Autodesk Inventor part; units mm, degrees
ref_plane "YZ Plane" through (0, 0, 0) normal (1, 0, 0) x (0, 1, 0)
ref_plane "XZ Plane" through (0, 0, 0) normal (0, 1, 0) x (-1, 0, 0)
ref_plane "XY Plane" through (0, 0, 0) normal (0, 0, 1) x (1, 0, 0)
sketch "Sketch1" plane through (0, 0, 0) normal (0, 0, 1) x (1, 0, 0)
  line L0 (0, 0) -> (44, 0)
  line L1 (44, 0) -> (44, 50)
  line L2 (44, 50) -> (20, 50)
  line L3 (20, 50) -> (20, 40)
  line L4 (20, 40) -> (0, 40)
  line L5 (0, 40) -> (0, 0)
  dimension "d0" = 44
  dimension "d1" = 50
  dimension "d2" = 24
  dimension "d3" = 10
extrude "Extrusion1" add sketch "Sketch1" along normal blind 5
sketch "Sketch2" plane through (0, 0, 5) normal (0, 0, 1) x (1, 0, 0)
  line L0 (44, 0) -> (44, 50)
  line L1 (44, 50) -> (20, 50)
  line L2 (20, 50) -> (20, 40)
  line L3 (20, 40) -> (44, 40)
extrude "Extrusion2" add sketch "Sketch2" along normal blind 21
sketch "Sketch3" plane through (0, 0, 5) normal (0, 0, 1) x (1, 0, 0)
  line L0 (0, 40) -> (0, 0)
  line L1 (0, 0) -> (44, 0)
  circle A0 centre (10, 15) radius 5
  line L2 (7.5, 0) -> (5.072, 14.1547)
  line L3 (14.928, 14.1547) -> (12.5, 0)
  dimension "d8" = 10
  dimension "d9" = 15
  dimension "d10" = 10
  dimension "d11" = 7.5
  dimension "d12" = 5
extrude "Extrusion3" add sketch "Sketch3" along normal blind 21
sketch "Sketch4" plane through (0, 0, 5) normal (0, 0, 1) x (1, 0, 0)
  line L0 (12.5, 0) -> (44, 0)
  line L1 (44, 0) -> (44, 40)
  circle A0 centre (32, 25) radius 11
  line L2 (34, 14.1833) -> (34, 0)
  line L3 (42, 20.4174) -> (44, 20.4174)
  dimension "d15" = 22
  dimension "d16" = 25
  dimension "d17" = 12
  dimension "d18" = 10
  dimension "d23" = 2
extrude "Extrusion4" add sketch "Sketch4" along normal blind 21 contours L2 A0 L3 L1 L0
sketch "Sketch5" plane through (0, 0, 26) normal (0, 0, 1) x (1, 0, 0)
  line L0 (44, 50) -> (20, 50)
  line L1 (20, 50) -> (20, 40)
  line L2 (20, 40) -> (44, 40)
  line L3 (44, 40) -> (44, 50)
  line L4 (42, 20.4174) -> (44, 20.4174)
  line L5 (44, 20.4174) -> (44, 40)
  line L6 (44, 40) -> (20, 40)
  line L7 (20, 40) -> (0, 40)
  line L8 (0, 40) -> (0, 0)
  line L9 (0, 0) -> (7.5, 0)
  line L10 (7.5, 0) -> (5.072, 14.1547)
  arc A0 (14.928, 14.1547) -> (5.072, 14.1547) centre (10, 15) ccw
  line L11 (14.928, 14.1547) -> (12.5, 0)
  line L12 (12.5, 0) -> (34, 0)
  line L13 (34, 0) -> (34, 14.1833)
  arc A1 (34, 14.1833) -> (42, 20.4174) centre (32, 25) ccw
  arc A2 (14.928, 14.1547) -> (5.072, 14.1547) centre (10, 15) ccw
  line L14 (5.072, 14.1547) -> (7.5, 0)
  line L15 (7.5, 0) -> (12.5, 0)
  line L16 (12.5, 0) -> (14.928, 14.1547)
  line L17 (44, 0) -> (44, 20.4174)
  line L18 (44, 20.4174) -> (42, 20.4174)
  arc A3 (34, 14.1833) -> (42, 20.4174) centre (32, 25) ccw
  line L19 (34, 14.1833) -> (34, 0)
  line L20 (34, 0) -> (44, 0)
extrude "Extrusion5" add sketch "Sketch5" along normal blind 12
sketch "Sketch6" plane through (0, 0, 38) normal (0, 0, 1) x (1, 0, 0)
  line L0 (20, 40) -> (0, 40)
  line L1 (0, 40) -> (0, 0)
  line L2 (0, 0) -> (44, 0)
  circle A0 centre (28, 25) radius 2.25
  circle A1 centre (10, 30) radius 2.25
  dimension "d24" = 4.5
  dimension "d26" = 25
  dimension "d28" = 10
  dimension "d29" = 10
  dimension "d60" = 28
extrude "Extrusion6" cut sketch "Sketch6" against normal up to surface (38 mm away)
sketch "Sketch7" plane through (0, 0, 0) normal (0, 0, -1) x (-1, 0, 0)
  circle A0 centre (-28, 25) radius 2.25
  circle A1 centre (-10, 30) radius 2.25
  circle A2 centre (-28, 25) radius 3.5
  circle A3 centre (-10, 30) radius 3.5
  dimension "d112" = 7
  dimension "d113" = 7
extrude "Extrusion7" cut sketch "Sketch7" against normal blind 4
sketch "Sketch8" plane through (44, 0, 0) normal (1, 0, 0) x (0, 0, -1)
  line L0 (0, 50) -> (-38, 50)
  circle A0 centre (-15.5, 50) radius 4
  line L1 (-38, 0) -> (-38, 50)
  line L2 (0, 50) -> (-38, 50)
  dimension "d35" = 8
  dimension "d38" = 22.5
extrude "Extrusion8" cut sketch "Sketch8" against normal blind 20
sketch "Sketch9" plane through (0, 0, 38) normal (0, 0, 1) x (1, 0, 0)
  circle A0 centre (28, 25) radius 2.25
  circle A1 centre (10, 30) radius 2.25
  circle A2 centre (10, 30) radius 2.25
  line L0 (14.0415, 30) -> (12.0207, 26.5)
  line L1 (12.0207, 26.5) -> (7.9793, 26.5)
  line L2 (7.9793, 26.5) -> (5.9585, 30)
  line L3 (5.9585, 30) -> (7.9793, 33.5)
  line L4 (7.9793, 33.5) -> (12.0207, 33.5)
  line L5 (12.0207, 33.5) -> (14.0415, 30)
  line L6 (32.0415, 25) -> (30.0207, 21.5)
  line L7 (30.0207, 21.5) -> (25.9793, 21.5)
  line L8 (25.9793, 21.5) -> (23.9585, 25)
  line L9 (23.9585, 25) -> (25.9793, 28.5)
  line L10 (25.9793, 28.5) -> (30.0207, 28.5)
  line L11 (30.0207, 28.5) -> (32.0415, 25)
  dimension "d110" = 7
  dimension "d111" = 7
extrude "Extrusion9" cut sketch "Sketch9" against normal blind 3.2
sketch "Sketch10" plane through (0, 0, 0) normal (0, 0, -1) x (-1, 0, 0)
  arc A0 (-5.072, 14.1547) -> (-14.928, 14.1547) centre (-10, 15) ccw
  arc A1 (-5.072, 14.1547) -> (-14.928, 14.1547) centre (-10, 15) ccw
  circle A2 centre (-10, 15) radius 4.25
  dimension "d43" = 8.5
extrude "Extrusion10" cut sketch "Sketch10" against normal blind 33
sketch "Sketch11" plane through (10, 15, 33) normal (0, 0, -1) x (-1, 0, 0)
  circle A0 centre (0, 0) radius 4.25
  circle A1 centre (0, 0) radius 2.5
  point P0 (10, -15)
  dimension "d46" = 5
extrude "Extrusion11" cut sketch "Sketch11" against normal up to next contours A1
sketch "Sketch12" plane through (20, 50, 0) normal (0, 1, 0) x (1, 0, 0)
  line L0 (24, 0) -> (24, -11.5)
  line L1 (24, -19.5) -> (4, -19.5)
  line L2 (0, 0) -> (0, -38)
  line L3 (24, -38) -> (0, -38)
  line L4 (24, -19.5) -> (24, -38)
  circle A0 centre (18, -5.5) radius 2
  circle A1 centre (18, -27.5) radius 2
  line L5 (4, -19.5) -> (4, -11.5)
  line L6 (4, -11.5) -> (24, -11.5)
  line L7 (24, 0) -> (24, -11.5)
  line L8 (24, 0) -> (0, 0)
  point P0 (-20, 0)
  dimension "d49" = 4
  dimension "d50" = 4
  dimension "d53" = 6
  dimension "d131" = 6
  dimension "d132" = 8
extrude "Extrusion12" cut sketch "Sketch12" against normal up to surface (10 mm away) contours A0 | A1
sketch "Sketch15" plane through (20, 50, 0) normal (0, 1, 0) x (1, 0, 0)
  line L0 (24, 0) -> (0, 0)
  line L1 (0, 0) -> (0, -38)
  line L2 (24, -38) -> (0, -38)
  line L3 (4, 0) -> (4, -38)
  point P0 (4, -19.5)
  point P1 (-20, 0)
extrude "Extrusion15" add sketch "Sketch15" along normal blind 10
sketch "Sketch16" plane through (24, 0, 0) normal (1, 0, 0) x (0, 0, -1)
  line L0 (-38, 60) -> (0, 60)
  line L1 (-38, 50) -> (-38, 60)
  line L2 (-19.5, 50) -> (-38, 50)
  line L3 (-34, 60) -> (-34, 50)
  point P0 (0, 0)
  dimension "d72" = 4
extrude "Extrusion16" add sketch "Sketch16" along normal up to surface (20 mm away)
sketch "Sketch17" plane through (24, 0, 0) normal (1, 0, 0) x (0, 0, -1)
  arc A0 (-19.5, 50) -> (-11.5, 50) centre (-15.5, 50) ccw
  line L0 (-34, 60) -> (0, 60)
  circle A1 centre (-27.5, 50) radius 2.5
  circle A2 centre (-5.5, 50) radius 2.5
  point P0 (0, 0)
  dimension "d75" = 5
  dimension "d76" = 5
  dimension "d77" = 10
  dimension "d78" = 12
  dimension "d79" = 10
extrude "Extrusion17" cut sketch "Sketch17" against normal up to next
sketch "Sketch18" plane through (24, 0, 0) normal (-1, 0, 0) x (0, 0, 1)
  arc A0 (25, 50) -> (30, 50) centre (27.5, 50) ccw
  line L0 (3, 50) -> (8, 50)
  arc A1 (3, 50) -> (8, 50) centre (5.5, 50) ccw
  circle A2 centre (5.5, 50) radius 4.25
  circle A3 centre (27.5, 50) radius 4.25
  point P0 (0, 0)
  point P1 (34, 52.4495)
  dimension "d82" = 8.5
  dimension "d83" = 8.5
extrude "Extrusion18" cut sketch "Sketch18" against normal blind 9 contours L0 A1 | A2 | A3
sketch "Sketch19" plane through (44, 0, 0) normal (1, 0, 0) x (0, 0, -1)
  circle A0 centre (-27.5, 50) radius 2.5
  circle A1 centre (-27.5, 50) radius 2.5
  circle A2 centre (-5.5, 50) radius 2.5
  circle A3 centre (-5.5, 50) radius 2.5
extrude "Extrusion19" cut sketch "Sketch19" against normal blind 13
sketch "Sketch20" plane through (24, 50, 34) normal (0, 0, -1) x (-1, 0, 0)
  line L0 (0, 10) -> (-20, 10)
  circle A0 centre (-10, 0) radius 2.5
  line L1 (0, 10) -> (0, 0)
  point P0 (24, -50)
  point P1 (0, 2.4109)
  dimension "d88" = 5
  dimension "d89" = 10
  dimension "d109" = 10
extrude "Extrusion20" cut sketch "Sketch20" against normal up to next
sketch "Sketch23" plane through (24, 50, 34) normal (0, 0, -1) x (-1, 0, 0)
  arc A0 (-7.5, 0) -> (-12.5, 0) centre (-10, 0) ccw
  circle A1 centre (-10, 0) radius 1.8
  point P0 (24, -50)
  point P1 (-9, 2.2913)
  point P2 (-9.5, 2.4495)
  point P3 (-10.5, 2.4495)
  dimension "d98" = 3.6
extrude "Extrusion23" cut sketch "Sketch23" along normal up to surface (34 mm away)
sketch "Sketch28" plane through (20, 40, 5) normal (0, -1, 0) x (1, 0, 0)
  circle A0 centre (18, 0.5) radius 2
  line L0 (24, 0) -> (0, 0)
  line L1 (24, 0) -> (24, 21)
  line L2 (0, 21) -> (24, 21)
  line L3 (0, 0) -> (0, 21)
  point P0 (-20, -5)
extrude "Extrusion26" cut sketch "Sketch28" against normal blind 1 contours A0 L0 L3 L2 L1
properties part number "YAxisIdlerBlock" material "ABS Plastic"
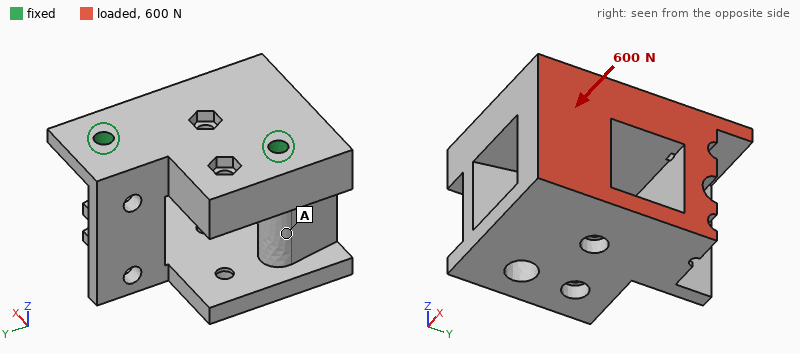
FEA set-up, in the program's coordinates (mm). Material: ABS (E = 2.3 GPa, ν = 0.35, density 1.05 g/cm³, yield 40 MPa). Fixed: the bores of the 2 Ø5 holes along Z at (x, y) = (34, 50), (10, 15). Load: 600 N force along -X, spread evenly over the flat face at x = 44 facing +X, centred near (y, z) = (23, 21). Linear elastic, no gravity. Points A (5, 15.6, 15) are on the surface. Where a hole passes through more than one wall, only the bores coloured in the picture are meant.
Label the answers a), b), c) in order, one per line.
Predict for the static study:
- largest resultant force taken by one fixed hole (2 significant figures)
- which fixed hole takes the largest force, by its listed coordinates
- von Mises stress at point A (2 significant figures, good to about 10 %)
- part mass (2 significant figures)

a) 420 N
b) (10, 15)
c) 4.6 MPa
d) 45 g
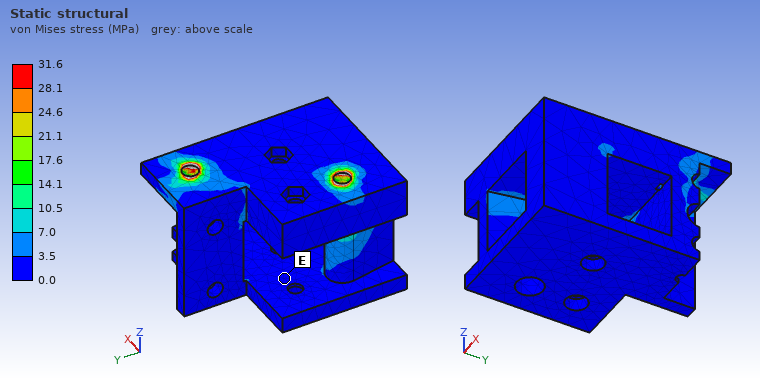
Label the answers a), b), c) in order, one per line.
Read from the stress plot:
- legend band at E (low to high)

a) 0.0 to 3.5 MPa
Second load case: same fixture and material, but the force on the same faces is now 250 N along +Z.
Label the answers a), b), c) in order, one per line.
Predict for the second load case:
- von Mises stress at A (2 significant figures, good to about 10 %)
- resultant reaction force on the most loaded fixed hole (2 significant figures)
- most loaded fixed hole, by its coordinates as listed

a) 2.7 MPa
b) 160 N
c) (34, 50)
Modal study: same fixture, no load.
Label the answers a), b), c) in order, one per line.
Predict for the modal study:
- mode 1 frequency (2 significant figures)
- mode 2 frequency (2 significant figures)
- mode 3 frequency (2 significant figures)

a) 630 Hz
b) 1600 Hz
c) 2100 Hz
